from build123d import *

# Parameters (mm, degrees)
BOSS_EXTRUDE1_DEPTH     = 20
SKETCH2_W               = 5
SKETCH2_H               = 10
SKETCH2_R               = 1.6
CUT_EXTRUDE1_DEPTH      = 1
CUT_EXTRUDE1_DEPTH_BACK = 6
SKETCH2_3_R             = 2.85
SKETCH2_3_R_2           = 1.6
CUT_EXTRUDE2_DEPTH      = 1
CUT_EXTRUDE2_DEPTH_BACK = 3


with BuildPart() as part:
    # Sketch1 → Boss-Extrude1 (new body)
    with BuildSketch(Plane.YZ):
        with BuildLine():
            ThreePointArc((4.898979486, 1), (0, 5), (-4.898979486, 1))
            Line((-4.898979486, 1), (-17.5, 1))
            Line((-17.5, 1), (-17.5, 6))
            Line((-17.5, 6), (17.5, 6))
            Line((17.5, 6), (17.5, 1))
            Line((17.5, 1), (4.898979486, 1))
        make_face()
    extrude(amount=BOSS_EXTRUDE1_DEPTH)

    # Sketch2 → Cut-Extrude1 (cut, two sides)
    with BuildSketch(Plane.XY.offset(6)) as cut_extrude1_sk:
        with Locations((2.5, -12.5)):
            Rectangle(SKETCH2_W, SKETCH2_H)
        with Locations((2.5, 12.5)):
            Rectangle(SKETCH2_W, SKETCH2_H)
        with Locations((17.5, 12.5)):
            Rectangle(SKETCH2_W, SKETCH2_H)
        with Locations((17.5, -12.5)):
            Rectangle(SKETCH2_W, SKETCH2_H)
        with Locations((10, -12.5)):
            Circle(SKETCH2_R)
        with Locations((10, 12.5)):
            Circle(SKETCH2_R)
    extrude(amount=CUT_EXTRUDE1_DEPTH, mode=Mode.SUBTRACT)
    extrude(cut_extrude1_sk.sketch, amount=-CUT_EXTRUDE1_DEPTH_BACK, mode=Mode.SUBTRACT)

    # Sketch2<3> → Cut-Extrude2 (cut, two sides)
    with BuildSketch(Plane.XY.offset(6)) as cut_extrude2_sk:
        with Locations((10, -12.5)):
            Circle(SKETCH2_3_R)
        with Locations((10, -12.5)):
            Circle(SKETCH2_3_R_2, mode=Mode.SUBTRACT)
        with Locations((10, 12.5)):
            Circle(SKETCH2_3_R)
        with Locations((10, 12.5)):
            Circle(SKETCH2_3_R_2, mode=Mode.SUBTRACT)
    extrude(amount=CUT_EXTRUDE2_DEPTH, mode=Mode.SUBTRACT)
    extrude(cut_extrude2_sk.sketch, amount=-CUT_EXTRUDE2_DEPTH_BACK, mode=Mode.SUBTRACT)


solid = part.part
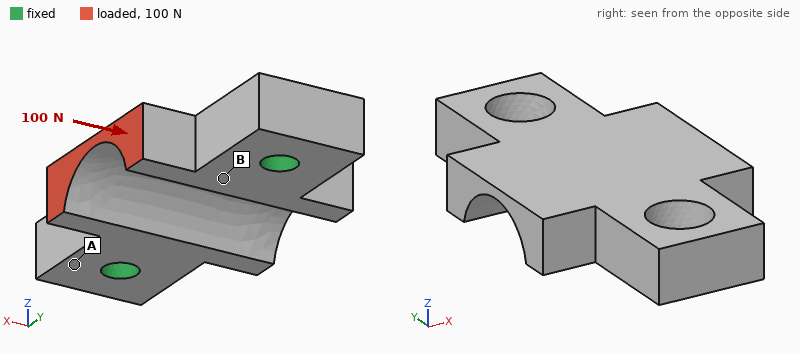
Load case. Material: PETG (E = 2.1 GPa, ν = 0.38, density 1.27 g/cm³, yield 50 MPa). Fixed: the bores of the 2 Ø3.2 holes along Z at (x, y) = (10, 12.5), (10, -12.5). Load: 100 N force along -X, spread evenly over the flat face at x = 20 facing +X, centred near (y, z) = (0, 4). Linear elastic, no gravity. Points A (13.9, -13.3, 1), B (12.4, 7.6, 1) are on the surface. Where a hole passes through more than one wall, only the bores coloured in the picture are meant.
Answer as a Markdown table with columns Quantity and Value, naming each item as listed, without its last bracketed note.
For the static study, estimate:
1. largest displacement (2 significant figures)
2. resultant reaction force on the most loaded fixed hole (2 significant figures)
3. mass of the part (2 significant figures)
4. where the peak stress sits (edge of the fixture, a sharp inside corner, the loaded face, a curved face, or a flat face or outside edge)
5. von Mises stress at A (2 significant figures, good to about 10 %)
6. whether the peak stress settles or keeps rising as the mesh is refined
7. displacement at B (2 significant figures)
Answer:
| Quantity | Value |
|---|---|
| largest displacement | 0.11 mm |
| resultant reaction force on the most loaded fixed hole | 50 N |
| mass of the part | 2.2 g |
| where the peak stress sits | edge of the fixture |
| von Mises stress at A | 2.9 MPa |
| whether the peak stress settles or keeps rising as the mesh is refined | keeps rising |
| displacement at B | 0.020 mm |
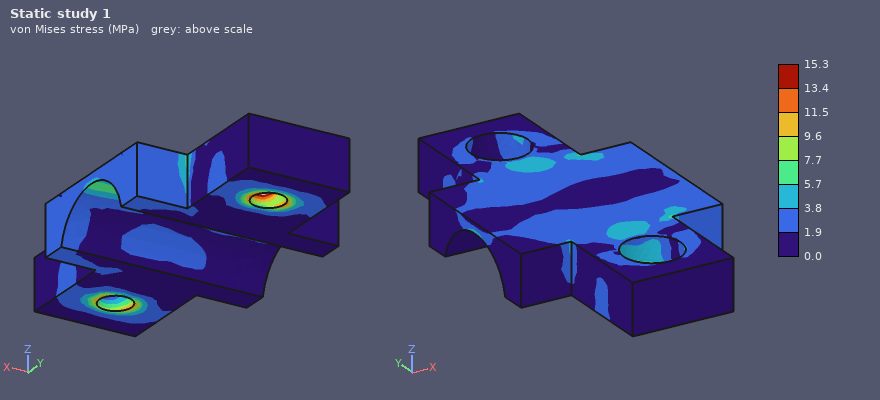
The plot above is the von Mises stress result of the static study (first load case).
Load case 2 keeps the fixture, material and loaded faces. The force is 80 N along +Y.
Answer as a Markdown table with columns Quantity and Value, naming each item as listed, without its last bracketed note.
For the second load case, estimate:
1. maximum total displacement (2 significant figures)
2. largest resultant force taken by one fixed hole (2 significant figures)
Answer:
| Quantity | Value |
|---|---|
| maximum total displacement | 92 µm |
| largest resultant force taken by one fixed hole | 50 N |
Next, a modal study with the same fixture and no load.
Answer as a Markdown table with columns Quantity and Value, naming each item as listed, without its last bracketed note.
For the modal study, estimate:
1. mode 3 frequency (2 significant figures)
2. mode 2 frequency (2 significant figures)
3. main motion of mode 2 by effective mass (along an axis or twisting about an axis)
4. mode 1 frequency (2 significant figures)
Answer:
| Quantity | Value |
|---|---|
| mode 3 frequency | 6400 Hz |
| mode 2 frequency | 6000 Hz |
| main motion of mode 2 by effective mass | along Z |
| mode 1 frequency | 3800 Hz |
